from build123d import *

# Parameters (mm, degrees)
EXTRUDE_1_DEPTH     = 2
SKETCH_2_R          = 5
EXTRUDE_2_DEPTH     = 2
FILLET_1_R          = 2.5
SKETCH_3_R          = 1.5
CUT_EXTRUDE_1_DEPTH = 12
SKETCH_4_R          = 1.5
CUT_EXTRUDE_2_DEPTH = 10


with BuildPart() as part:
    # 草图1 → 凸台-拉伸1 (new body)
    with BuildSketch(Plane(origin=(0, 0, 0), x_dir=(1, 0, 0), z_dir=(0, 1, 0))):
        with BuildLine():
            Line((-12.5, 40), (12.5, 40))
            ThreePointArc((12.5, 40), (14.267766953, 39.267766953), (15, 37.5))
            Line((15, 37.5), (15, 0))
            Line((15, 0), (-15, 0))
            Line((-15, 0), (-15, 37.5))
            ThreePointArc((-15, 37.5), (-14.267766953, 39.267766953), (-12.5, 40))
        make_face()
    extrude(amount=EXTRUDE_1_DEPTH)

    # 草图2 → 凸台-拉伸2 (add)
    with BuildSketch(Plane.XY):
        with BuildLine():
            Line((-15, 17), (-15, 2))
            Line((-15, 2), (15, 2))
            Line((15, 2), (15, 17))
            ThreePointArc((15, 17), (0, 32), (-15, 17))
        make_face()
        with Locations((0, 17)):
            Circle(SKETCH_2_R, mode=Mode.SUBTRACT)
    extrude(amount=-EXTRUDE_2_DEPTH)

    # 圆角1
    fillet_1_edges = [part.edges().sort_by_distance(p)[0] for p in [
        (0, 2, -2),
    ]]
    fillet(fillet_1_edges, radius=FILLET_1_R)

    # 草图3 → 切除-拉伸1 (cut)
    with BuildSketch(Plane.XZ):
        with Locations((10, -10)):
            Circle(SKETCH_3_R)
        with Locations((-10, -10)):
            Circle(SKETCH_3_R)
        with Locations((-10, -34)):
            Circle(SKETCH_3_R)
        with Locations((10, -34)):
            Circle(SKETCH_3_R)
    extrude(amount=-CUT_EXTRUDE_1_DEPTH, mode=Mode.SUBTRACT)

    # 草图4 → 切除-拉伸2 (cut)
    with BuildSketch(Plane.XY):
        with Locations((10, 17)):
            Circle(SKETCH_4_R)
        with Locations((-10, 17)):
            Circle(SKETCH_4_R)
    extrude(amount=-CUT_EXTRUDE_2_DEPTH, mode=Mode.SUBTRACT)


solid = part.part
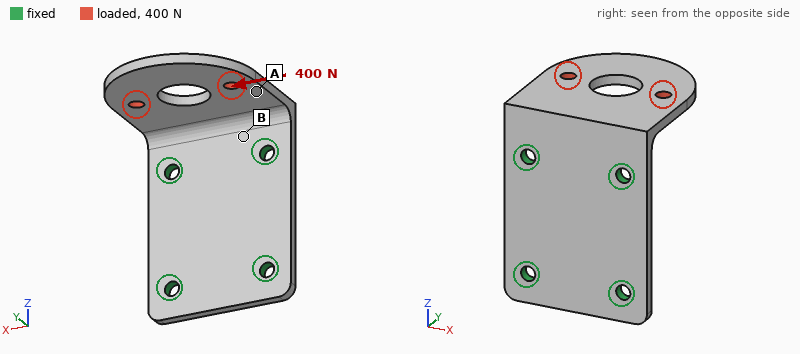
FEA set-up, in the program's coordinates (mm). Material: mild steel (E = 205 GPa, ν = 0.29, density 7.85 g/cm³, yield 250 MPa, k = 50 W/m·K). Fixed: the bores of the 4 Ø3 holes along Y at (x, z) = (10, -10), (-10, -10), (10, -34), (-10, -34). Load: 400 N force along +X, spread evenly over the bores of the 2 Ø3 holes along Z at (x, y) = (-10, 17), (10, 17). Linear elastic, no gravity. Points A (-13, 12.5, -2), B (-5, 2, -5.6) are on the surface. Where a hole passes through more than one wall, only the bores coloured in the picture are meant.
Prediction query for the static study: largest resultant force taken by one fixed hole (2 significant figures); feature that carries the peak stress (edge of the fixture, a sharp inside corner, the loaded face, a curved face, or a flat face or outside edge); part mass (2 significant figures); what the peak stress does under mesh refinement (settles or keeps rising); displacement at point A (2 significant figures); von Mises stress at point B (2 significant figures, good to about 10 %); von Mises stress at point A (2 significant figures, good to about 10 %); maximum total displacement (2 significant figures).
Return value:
390 N
edge of the fixture
30 g
keeps rising
35 µm
78 MPa
32 MPa
55 µm
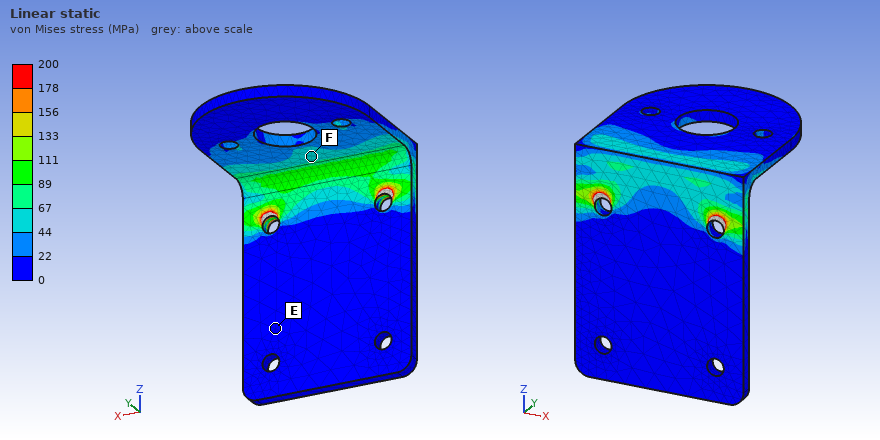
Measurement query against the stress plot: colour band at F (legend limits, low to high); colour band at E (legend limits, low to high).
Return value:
44 to 67 MPa
0 to 22 MPa
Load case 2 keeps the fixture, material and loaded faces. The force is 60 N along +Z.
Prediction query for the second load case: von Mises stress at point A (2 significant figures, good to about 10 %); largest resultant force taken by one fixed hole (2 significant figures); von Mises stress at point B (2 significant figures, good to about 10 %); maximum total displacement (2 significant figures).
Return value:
15 MPa
26 N
42 MPa
89 µm
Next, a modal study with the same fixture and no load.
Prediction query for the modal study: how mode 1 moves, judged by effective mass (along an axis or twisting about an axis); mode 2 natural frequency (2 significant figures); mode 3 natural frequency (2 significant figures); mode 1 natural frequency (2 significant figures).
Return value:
along Z
4200 Hz
6200 Hz
1600 Hz
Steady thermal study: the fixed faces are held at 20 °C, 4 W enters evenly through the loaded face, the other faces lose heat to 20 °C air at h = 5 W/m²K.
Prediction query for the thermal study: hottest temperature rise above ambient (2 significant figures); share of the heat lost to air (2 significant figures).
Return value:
38 K
6.3 %
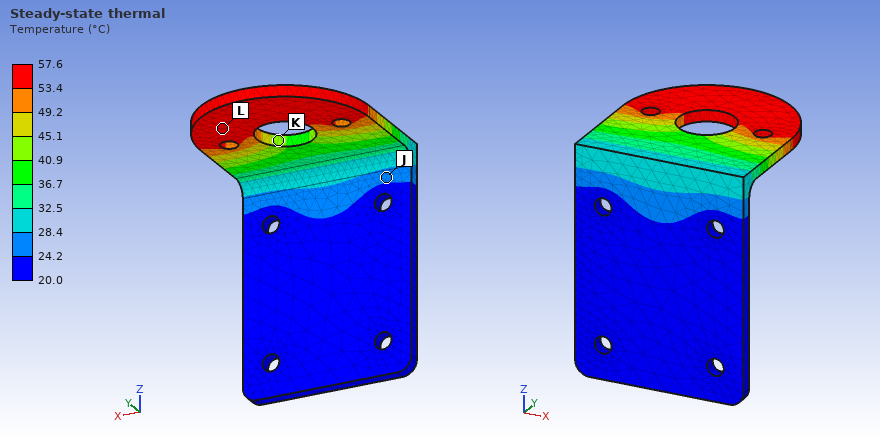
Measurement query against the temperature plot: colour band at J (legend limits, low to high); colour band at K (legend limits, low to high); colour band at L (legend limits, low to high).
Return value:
24.2 to 28.4 °C
40.9 to 45.1 °C
53.4 to 57.6 °C
